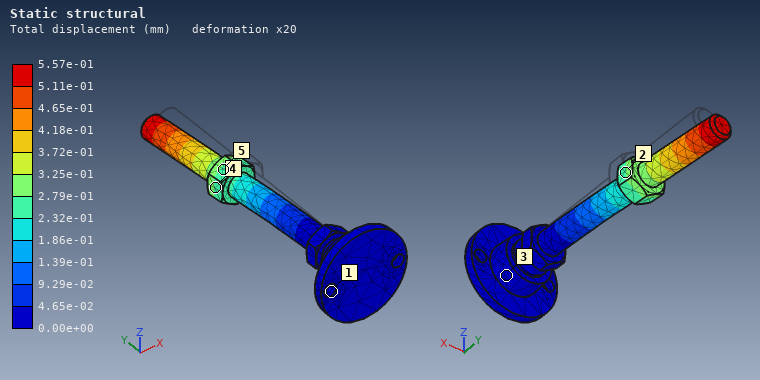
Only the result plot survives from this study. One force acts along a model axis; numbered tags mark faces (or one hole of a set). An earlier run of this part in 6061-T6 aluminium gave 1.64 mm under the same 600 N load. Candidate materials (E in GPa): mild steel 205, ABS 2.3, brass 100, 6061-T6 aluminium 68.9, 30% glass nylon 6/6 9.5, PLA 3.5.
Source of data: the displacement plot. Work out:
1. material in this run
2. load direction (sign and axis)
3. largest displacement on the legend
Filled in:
mild steel
-X
5.57e-01 mm
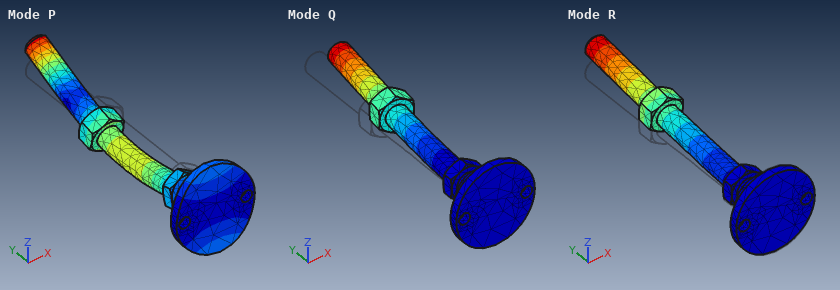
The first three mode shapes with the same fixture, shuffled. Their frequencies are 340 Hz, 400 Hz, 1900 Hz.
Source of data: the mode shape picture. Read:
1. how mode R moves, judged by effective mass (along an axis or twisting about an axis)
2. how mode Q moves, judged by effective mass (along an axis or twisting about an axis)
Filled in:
along Z
along X
